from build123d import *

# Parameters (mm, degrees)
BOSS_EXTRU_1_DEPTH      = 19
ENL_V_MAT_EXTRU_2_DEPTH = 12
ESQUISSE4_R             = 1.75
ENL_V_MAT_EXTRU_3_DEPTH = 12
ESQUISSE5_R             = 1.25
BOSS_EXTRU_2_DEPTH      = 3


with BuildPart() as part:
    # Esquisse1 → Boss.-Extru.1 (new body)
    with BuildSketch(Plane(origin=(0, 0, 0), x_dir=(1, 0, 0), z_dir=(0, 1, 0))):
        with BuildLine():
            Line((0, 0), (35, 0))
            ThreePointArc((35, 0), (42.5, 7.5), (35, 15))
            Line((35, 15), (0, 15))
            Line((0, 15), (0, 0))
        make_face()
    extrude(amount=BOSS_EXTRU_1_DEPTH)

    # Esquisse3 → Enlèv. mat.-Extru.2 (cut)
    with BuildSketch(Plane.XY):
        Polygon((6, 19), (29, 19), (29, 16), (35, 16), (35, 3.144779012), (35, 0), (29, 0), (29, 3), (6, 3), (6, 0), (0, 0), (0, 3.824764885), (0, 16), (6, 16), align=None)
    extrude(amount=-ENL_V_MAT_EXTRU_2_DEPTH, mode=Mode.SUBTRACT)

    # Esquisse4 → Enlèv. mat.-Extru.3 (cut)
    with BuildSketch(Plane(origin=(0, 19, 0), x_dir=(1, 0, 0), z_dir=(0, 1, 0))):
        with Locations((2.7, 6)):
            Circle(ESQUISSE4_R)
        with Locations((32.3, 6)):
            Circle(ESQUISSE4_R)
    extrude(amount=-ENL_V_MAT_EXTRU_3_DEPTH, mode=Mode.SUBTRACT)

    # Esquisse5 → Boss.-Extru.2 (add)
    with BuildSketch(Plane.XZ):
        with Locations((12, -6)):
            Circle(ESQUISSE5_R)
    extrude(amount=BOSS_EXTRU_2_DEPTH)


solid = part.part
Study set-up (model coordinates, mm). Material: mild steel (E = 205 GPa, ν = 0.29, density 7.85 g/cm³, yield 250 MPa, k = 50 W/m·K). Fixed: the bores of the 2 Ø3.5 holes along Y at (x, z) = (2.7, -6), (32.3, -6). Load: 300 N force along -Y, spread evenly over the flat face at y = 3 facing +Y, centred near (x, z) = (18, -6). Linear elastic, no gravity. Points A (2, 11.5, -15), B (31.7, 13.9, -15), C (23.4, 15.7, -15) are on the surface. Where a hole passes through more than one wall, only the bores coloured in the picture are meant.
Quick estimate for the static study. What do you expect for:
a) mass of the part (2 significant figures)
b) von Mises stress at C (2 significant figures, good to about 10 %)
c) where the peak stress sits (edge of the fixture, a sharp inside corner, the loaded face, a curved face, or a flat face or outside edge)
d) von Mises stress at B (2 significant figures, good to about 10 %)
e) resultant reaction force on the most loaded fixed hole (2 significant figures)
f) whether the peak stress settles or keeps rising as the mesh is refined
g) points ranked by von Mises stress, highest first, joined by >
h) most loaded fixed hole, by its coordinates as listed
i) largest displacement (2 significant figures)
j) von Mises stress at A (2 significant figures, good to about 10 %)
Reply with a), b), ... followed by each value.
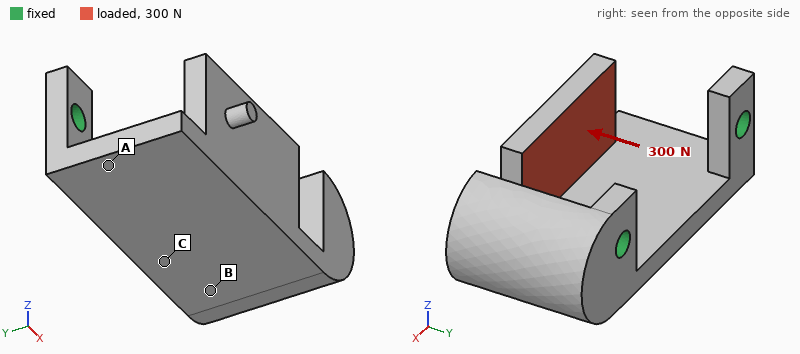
a) 38 g
b) 17 MPa
c) a sharp inside corner
d) 7.3 MPa
e) 160 N
f) keeps rising
g) A > C > B
h) (2.7, -6)
i) 42 µm
j) 32 MPa
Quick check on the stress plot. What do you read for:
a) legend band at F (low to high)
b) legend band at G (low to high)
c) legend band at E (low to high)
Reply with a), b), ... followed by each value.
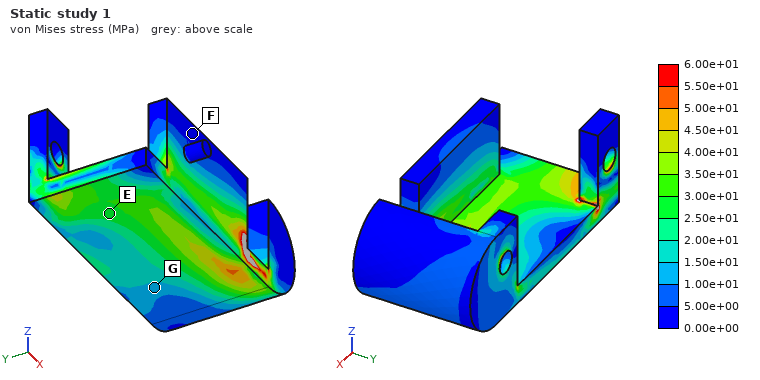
a) 0.00e+00 to 5.00e+00 MPa
b) 1.00e+01 to 1.50e+01 MPa
c) 2.50e+01 to 3.00e+01 MPa
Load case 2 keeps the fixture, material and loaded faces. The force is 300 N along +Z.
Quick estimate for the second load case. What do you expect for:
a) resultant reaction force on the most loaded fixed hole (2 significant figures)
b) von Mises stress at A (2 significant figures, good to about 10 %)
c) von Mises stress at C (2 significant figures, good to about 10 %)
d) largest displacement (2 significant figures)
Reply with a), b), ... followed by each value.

a) 160 N
b) 36 MPa
c) 29 MPa
d) 61 µm
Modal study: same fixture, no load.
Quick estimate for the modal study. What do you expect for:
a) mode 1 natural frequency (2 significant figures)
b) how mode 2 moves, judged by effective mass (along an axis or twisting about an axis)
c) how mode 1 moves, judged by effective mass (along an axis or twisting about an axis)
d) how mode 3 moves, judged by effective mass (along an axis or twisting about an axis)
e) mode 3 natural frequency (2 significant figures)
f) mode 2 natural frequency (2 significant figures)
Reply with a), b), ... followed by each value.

a) 3400 Hz
b) along X
c) along Z
d) along Y
e) 7800 Hz
f) 5900 Hz
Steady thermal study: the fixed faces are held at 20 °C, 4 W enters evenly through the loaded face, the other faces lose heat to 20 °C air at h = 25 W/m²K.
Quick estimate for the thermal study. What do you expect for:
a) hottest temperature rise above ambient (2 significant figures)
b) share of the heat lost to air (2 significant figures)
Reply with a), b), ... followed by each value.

a) 26 K
b) 21 %
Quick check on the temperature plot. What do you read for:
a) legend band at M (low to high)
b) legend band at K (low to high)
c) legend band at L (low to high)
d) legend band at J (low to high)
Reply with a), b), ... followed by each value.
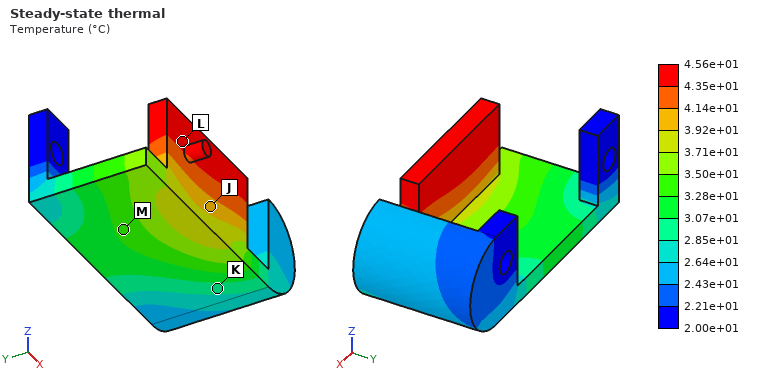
a) 3.28e+01 to 3.50e+01 °C
b) 2.85e+01 to 3.07e+01 °C
c) 4.35e+01 to 4.56e+01 °C
d) 3.92e+01 to 4.14e+01 °C
